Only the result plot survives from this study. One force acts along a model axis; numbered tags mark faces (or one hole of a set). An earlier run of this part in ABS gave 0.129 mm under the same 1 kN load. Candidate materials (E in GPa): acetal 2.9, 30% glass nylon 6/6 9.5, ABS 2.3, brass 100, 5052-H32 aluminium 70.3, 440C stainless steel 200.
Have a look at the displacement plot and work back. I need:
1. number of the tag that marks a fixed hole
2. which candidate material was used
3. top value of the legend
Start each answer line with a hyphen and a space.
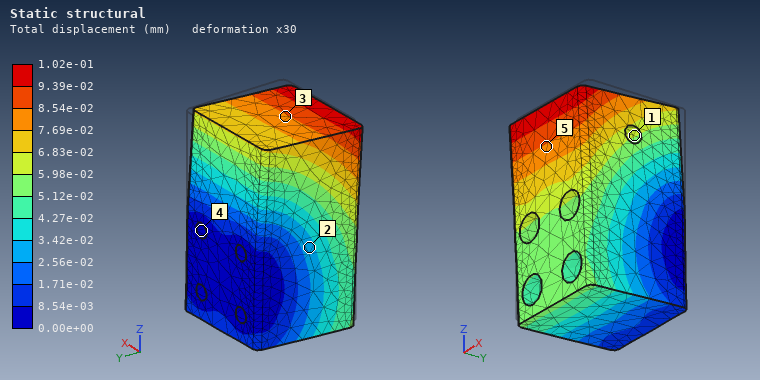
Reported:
- 4
- acetal
- 1.02e-01 mm
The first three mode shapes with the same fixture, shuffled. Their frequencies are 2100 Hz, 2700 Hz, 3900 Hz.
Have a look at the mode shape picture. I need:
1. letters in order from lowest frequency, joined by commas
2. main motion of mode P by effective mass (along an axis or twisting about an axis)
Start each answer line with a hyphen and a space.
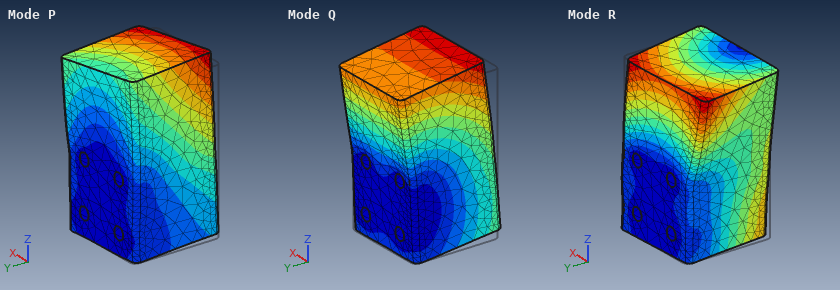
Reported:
- Q, P, R
- along X
